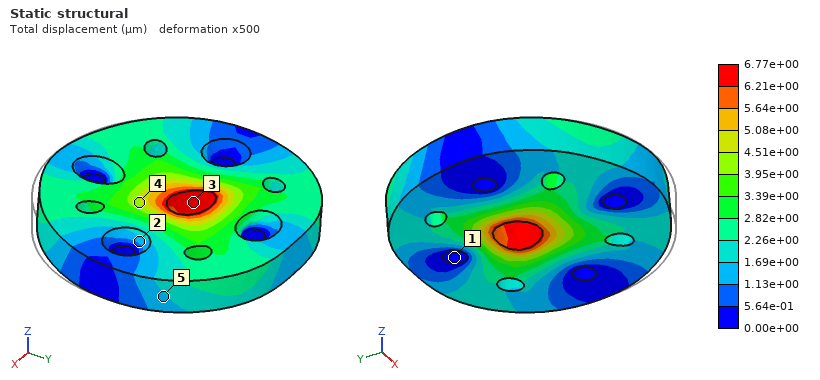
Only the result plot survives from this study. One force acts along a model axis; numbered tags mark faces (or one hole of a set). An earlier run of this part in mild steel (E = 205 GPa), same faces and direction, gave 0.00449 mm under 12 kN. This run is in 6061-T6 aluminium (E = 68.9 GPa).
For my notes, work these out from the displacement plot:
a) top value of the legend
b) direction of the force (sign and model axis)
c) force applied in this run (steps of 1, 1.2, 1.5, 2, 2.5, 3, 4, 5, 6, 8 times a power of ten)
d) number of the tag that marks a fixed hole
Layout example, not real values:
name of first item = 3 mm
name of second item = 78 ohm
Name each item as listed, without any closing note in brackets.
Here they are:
top value of the legend = 6.77e+00 µm
direction of the force = +Y
force applied in this run = 6 kN
number of the tag that marks a fixed hole = 1
